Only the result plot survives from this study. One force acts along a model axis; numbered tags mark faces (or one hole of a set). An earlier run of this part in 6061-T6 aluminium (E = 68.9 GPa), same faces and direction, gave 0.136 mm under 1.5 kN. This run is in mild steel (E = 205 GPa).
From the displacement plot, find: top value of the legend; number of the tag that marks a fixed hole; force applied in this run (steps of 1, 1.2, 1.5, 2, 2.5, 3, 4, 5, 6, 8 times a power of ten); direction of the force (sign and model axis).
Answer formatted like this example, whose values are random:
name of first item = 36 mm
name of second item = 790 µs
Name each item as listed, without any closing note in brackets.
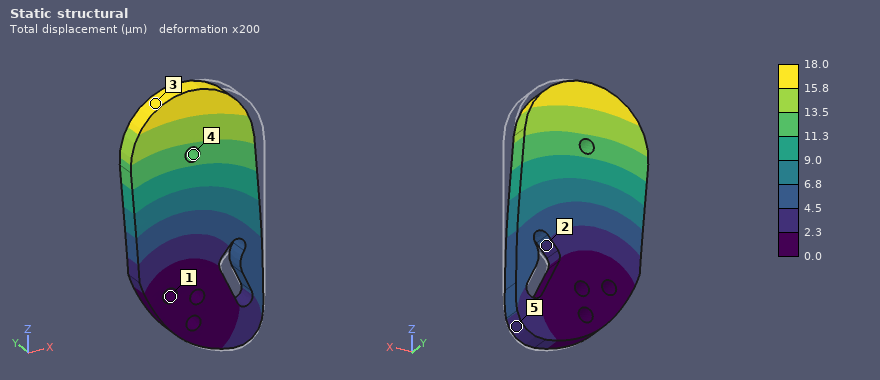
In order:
top value of the legend = 18.0 µm
number of the tag that marks a fixed hole = 1
force applied in this run = 600 N
direction of the force = -X
